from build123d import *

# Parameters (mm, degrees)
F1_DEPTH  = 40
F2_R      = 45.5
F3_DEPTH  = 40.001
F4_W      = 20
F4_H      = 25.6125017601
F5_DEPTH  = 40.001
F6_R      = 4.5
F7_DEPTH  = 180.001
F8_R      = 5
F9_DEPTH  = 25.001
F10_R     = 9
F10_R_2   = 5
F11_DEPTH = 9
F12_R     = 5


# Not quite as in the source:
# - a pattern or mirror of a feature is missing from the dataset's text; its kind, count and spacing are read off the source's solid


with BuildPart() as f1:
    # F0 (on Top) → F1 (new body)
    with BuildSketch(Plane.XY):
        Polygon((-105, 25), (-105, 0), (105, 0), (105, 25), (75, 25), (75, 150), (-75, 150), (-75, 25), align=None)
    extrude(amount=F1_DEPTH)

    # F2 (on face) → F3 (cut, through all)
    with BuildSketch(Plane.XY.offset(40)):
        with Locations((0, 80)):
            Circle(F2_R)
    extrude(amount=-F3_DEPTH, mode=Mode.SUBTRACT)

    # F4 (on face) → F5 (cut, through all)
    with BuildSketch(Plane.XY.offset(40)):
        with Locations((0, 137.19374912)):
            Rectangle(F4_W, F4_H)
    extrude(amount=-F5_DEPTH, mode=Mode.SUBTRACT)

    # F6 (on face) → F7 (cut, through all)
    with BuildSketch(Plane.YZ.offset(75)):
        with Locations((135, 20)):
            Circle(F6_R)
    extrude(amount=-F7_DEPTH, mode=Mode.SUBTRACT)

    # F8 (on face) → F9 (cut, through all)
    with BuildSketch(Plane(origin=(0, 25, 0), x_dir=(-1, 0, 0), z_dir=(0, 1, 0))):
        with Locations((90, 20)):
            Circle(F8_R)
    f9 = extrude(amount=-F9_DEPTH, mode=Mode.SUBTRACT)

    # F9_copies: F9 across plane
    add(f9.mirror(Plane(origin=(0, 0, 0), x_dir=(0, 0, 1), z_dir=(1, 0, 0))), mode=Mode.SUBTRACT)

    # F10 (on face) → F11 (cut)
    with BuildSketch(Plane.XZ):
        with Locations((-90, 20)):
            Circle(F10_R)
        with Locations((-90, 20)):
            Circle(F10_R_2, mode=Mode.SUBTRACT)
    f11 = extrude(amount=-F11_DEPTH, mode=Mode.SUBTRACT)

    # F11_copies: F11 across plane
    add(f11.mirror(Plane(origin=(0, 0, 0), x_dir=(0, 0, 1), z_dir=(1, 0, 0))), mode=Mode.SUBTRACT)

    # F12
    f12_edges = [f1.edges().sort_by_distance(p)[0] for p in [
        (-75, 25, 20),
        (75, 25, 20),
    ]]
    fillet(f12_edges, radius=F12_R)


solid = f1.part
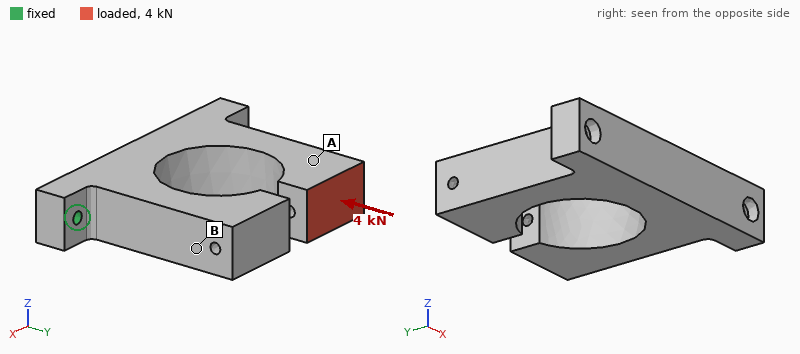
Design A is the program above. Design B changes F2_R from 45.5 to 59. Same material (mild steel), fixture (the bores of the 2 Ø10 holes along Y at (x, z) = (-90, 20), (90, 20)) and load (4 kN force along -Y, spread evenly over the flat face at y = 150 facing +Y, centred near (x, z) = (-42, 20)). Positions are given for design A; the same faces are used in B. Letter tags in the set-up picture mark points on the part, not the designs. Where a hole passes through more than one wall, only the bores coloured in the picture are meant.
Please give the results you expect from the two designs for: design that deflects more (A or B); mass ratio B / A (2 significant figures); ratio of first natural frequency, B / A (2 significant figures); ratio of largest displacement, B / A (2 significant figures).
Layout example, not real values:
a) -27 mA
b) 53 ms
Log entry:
a) B
b) 0.75
c) 0.95
d) 5.8
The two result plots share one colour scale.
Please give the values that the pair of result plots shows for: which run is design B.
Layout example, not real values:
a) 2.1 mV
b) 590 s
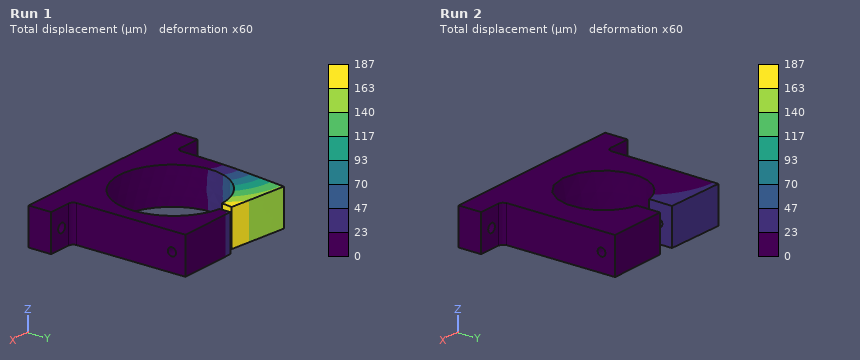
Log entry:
a) Run 1
